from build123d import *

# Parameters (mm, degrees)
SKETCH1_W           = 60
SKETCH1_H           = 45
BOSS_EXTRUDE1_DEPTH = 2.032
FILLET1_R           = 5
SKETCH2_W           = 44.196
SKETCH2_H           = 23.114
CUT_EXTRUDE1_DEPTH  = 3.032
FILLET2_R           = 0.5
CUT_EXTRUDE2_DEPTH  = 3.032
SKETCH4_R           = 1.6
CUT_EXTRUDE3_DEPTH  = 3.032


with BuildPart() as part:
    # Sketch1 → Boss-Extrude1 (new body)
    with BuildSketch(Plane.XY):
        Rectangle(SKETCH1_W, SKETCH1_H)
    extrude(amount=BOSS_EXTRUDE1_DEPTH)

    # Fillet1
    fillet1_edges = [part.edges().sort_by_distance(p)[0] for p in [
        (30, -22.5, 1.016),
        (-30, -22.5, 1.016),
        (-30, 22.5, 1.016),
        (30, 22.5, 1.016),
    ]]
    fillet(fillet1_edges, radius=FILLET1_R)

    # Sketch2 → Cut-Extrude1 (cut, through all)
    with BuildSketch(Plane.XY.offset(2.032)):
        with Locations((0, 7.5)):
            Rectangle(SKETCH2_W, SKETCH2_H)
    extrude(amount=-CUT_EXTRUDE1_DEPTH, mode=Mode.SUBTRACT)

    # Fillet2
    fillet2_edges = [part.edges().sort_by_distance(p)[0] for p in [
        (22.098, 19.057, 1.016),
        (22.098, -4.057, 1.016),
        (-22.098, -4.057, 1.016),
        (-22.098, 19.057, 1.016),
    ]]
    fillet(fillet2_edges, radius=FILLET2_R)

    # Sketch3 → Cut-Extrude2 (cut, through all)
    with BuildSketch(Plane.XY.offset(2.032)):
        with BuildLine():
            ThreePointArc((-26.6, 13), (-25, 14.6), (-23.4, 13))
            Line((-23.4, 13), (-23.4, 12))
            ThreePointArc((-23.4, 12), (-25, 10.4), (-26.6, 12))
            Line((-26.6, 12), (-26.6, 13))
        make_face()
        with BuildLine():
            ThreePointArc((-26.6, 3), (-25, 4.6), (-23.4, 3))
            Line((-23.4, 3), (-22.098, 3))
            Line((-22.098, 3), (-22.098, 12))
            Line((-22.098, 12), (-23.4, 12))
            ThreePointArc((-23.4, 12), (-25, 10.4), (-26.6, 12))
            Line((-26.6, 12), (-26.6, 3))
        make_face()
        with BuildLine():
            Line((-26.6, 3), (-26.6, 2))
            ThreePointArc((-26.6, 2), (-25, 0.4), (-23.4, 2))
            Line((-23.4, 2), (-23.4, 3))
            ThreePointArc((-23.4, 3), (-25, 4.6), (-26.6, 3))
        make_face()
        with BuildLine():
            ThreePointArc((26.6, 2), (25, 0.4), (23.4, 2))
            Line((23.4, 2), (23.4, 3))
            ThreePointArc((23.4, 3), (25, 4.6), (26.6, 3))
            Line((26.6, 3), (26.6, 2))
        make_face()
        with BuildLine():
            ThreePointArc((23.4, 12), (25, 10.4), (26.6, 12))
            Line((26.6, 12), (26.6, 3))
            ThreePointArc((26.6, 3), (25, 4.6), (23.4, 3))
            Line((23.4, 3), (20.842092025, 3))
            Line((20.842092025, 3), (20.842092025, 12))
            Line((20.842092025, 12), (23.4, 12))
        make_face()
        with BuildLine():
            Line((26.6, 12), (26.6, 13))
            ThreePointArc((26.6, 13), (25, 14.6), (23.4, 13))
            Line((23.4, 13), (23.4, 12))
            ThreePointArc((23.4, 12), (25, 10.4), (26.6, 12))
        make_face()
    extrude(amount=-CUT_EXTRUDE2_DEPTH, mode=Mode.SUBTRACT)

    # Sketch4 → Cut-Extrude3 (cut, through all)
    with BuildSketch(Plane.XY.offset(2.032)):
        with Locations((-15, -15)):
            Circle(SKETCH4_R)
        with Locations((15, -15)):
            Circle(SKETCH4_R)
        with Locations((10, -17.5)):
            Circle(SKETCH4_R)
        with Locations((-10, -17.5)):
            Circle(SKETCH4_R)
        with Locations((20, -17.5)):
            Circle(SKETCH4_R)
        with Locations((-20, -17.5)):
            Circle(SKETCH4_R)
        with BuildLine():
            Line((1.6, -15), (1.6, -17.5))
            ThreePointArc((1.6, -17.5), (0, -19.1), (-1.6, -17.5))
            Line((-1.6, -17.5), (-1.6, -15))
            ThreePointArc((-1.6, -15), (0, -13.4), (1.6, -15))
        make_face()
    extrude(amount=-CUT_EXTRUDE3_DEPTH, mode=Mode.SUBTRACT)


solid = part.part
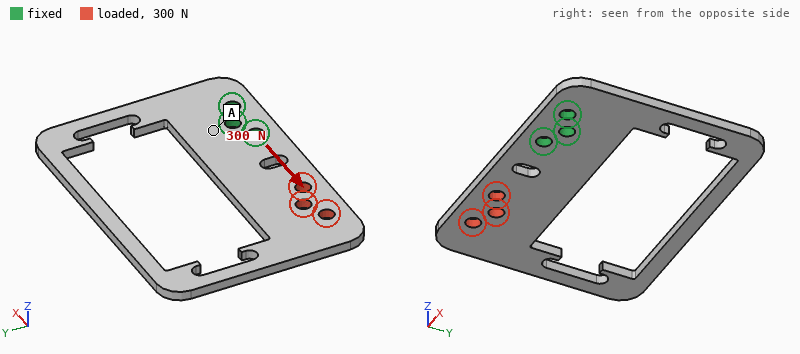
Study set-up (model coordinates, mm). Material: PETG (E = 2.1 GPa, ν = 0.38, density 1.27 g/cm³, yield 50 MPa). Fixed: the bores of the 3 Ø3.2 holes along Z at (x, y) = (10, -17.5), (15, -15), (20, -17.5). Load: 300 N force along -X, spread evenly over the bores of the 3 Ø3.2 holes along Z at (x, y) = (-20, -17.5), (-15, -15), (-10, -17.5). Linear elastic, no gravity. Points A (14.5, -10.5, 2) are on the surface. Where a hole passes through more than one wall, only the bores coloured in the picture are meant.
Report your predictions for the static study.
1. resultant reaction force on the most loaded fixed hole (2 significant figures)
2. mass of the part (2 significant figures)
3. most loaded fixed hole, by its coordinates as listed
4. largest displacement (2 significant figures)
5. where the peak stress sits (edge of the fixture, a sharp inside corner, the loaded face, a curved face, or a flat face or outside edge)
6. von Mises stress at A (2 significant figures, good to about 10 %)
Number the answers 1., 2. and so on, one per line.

1. 210 N
2. 3.8 g
3. (10, -17.5)
4. 0.40 mm
5. a curved face
6. 2.7 MPa
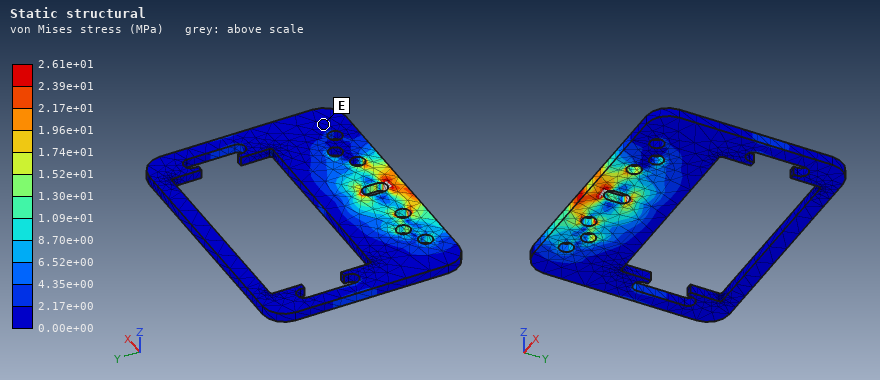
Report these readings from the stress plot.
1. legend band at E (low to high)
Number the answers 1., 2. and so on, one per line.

1. 0.00e+00 to 2.17e+00 MPa
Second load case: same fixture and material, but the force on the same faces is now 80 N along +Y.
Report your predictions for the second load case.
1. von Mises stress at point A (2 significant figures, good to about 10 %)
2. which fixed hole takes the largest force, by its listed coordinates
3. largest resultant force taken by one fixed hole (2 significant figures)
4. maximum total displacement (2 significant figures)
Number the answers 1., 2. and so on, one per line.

1. 8.8 MPa
2. (10, -17.5)
3. 220 N
4. 0.89 mm
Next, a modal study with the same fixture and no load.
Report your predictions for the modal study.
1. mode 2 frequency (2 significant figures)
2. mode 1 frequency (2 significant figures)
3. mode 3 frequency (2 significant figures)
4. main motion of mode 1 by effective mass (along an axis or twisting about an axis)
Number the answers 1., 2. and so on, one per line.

1. 250 Hz
2. 150 Hz
3. 420 Hz
4. along Z
